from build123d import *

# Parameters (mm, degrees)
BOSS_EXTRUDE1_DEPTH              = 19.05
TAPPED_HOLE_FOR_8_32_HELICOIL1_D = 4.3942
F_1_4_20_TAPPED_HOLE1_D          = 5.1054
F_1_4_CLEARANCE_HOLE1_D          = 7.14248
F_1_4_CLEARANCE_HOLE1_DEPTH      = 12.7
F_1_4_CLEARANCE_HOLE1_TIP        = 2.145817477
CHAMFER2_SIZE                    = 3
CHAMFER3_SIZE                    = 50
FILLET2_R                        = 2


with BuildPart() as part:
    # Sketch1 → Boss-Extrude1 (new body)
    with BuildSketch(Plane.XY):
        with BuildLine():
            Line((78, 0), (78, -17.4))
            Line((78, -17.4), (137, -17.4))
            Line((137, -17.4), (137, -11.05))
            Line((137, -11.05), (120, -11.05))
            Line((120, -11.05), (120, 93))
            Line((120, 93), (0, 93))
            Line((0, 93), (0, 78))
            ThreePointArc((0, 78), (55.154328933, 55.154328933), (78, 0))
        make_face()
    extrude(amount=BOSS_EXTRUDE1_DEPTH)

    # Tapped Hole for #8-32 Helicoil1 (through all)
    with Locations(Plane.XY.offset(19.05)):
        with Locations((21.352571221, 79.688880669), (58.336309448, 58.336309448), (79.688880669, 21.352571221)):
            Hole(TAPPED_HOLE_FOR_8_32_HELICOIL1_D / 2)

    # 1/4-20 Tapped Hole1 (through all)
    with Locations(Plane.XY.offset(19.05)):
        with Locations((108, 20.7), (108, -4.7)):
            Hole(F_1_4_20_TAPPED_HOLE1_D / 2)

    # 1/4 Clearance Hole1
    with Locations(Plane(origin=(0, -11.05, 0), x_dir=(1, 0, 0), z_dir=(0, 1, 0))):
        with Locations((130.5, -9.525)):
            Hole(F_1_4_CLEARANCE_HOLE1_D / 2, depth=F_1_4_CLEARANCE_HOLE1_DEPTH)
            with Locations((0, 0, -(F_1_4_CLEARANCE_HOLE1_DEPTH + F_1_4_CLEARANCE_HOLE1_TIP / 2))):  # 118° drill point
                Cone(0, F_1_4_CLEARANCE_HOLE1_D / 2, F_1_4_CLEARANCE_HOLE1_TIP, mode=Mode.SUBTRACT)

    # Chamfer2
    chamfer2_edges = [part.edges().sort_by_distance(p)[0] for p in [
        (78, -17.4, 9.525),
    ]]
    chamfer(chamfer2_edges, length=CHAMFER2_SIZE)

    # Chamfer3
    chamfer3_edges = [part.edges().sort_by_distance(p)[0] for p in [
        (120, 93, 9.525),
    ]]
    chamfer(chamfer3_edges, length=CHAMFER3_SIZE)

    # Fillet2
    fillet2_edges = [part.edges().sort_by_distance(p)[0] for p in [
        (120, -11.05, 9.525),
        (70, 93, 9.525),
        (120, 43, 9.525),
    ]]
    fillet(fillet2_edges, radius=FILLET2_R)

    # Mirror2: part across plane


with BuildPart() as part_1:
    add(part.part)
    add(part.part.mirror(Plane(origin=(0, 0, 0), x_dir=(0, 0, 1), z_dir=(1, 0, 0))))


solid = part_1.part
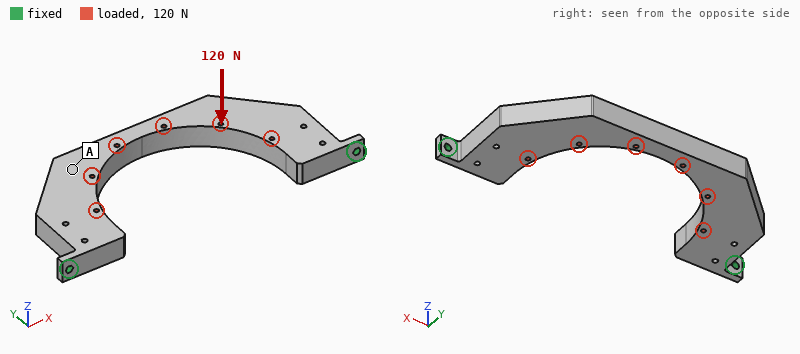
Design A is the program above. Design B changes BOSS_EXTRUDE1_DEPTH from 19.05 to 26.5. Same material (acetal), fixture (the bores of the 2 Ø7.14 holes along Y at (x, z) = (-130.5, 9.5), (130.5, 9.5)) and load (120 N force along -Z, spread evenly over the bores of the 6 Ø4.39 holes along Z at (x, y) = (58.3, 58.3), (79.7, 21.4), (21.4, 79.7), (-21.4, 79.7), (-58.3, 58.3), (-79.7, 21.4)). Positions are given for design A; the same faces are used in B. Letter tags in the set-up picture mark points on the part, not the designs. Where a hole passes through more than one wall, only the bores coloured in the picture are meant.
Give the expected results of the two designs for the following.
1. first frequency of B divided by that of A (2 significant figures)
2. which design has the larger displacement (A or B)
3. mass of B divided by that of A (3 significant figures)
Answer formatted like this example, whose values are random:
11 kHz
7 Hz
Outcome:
1.0
A
1.39
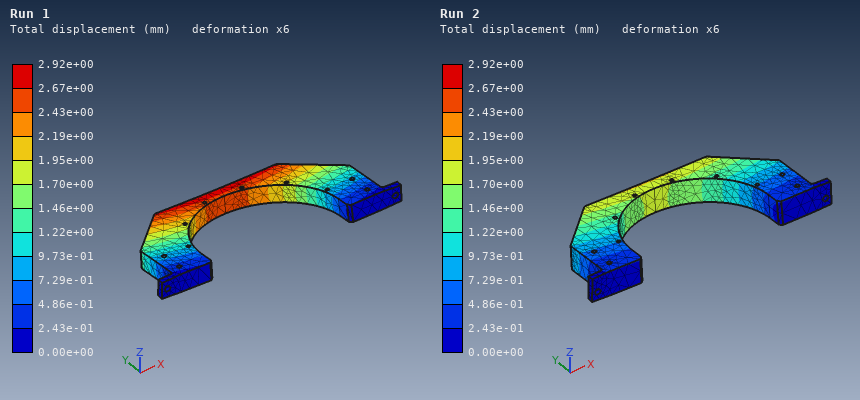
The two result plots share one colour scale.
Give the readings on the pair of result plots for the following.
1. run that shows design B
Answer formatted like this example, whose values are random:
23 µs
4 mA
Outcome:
Run 2
